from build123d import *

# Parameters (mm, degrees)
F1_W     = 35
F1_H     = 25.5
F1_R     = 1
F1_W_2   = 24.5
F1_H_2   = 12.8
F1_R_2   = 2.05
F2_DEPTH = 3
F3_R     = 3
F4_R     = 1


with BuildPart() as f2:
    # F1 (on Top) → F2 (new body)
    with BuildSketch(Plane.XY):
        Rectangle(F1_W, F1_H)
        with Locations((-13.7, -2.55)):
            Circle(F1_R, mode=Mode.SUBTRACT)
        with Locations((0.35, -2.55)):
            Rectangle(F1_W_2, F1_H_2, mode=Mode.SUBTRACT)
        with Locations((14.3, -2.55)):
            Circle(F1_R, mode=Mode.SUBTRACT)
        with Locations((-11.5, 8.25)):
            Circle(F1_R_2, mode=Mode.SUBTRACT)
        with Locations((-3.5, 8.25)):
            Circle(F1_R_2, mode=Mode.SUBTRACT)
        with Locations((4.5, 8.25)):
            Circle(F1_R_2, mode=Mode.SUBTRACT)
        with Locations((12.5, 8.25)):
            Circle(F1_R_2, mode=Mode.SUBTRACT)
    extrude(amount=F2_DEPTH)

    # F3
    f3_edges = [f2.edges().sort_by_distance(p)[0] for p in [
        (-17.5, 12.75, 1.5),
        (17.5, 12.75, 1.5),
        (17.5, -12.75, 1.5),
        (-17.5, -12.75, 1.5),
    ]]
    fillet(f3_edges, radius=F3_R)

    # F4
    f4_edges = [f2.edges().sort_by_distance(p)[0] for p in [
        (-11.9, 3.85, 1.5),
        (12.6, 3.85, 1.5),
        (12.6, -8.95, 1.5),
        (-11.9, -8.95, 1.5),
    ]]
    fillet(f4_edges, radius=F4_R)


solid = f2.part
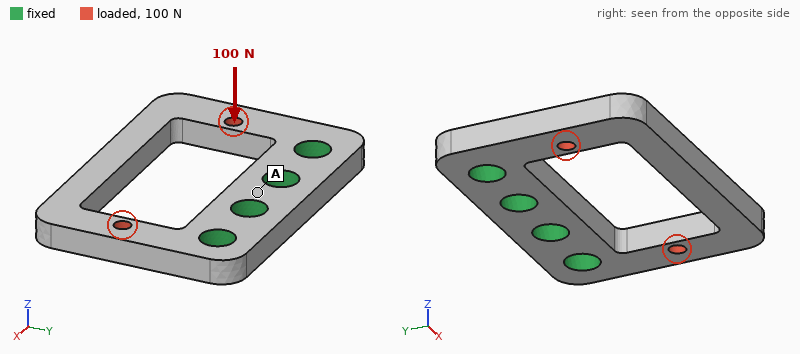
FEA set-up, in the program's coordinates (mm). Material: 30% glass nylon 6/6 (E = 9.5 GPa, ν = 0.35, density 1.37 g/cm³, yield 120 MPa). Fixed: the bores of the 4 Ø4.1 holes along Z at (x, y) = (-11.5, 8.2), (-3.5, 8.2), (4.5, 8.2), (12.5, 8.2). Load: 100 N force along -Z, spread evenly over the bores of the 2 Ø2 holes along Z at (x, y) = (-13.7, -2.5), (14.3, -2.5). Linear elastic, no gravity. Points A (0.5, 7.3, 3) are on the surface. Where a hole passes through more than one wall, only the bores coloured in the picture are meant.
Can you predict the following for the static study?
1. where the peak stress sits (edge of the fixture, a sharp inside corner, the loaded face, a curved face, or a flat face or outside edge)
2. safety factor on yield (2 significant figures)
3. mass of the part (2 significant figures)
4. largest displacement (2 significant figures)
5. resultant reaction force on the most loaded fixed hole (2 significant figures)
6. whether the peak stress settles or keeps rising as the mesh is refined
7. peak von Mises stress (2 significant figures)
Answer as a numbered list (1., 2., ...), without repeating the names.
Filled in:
1. a curved face
2. 1.6
3. 2.1 g
4. 0.33 mm
5. 54 N
6. settles
7. 75 MPa
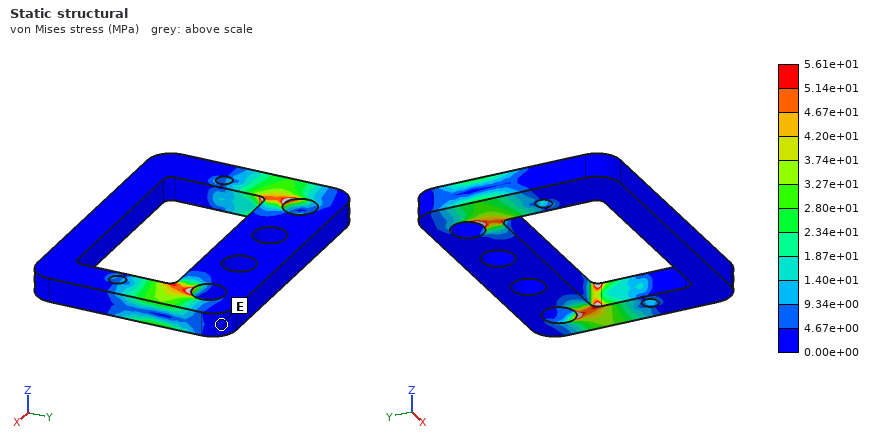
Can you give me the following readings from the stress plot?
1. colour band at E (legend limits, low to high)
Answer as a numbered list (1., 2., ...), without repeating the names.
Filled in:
1. 0.00e+00 to 4.67e+00 MPa
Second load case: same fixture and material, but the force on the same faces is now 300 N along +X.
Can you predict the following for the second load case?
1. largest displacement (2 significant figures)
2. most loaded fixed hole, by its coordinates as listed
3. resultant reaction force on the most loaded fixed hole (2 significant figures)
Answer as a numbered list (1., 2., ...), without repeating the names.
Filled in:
1. 0.20 mm
2. (-11.5, 8.2)
3. 130 N
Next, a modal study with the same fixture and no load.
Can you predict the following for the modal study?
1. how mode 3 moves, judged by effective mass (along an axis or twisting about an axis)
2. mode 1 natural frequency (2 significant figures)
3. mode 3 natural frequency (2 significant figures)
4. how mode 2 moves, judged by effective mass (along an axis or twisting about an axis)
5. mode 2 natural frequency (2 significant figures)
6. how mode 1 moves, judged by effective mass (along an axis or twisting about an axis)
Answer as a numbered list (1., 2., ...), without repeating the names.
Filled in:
1. along X
2. 2100 Hz
3. 5000 Hz
4. twisting about Y
5. 3800 Hz
6. along Z
